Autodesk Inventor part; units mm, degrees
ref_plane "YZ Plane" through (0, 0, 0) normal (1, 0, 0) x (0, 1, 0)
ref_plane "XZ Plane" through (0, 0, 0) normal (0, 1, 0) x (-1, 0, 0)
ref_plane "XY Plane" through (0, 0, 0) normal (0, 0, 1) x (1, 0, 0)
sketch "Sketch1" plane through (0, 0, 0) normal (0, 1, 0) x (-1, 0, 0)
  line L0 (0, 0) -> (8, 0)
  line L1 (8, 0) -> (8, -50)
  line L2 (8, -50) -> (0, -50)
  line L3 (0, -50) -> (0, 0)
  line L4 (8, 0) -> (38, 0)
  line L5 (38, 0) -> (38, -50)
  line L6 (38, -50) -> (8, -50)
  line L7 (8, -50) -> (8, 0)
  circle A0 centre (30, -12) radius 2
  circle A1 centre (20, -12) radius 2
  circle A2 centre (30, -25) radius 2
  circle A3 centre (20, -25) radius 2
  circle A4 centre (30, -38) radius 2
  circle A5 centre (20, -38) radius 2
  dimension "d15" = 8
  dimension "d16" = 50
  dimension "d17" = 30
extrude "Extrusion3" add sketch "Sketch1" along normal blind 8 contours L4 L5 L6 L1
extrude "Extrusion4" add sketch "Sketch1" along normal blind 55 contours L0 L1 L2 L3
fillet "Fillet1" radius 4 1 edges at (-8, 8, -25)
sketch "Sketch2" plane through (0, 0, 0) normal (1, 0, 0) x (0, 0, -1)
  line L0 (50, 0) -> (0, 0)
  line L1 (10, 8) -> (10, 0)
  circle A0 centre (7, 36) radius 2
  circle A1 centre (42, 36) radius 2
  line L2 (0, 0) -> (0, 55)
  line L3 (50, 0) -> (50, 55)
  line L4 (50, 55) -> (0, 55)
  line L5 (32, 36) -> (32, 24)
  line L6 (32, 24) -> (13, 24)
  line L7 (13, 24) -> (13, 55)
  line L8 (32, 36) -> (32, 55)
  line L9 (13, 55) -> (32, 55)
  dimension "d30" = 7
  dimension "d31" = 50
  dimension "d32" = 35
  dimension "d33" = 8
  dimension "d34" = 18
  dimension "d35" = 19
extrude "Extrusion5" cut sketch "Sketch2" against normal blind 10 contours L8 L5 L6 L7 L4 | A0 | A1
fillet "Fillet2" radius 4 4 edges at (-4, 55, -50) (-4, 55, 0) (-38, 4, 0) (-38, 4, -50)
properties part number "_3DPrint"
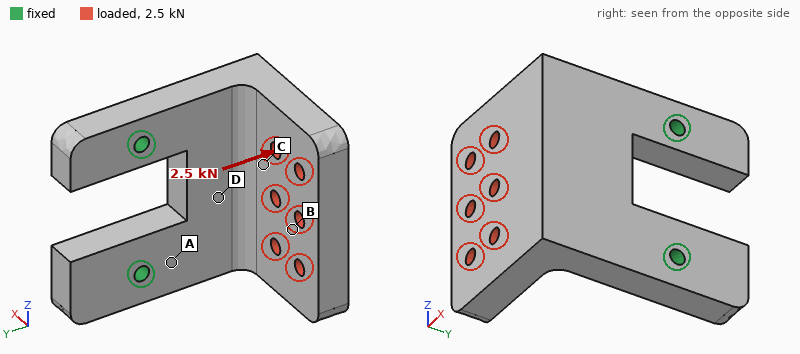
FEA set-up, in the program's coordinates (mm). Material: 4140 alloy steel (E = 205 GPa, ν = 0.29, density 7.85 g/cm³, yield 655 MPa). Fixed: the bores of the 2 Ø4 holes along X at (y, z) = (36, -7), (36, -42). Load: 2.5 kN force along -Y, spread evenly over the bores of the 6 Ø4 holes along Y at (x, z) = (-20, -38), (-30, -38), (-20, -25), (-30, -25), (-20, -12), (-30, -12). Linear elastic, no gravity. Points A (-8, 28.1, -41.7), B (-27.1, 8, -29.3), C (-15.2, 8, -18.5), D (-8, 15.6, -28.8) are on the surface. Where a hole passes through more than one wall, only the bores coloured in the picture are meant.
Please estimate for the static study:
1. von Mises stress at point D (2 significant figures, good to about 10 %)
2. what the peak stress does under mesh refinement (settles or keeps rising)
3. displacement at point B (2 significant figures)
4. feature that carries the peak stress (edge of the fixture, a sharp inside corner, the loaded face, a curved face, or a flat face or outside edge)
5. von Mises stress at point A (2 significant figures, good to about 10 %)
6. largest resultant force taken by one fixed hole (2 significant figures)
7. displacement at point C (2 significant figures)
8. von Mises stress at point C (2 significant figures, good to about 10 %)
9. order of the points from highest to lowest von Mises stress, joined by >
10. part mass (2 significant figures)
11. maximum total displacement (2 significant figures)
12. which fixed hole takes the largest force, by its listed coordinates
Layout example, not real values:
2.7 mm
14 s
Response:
80 MPa
keeps rising
0.14 mm
edge of the fixture
170 MPa
1.4 kN
0.092 mm
50 MPa
A > D > C > B
220 g
0.22 mm
(36, -42)
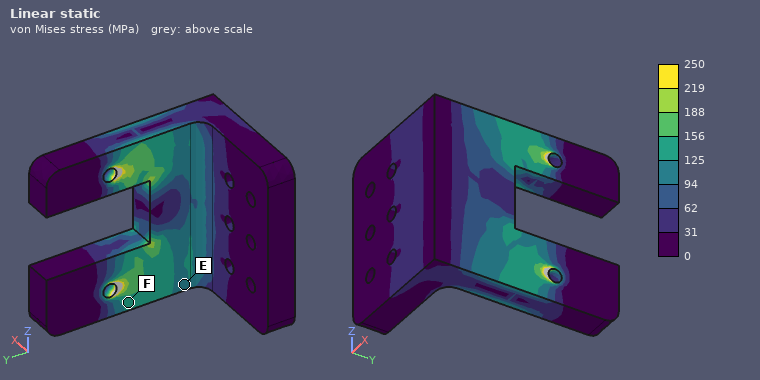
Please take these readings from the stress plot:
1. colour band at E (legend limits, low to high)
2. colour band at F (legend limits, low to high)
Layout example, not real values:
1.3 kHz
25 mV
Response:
94 to 125 MPa
125 to 156 MPa
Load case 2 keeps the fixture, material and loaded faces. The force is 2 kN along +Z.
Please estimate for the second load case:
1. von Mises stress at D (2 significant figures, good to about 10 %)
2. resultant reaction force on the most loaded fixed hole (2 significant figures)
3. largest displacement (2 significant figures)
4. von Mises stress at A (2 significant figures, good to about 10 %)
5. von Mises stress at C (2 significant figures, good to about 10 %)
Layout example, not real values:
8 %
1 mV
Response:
62 MPa
2.1 kN
55 µm
55 MPa
26 MPa
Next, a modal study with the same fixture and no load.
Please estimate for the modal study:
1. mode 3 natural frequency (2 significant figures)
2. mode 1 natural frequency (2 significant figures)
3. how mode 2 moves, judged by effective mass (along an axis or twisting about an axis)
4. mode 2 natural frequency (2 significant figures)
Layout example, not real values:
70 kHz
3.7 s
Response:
5700 Hz
1700 Hz
along Z
3500 Hz
